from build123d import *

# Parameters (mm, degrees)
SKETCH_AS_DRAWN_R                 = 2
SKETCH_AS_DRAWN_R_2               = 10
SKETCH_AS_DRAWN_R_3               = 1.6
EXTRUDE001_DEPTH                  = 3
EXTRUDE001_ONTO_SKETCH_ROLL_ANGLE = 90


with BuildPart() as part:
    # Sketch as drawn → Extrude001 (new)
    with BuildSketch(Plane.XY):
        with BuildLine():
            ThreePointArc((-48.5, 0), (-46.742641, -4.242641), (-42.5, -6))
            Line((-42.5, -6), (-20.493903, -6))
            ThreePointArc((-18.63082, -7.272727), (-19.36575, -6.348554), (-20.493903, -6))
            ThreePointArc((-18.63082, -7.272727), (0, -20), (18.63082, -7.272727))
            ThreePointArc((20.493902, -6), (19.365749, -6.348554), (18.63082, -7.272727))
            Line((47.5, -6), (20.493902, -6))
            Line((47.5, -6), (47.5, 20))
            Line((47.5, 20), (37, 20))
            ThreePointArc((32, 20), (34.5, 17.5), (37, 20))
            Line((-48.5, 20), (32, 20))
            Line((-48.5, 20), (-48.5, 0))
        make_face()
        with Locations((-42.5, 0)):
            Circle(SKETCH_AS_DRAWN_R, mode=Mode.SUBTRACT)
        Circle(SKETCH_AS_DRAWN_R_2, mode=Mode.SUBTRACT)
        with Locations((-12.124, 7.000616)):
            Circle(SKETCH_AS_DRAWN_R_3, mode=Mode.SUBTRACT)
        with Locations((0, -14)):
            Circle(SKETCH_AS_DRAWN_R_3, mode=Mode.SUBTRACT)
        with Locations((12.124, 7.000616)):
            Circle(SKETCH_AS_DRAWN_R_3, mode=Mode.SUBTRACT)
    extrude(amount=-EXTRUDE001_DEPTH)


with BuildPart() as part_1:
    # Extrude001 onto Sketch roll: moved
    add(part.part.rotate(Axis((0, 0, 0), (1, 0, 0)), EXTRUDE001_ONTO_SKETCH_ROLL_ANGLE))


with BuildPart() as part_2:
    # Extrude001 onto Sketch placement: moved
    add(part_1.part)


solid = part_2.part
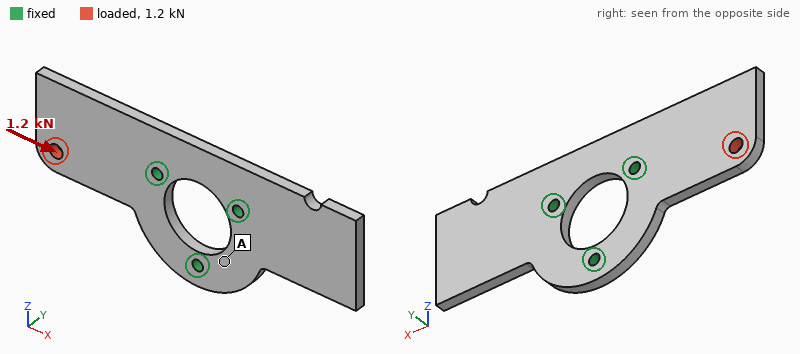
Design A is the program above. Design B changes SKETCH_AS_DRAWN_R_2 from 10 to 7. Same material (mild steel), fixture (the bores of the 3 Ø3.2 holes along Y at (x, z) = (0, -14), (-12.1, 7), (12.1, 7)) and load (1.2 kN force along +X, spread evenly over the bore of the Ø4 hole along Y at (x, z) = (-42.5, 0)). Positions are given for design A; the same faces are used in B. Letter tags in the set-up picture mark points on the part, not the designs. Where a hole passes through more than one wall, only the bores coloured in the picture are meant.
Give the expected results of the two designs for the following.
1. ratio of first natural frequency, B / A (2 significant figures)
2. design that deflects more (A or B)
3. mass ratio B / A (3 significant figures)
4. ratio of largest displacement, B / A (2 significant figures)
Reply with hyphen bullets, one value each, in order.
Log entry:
- 1.0
- A
- 1.06
- 0.91
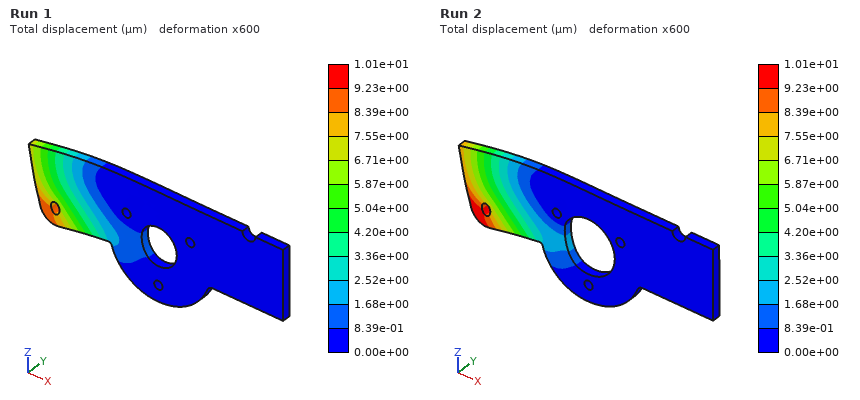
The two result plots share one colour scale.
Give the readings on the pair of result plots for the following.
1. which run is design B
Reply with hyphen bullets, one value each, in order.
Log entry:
- Run 1
